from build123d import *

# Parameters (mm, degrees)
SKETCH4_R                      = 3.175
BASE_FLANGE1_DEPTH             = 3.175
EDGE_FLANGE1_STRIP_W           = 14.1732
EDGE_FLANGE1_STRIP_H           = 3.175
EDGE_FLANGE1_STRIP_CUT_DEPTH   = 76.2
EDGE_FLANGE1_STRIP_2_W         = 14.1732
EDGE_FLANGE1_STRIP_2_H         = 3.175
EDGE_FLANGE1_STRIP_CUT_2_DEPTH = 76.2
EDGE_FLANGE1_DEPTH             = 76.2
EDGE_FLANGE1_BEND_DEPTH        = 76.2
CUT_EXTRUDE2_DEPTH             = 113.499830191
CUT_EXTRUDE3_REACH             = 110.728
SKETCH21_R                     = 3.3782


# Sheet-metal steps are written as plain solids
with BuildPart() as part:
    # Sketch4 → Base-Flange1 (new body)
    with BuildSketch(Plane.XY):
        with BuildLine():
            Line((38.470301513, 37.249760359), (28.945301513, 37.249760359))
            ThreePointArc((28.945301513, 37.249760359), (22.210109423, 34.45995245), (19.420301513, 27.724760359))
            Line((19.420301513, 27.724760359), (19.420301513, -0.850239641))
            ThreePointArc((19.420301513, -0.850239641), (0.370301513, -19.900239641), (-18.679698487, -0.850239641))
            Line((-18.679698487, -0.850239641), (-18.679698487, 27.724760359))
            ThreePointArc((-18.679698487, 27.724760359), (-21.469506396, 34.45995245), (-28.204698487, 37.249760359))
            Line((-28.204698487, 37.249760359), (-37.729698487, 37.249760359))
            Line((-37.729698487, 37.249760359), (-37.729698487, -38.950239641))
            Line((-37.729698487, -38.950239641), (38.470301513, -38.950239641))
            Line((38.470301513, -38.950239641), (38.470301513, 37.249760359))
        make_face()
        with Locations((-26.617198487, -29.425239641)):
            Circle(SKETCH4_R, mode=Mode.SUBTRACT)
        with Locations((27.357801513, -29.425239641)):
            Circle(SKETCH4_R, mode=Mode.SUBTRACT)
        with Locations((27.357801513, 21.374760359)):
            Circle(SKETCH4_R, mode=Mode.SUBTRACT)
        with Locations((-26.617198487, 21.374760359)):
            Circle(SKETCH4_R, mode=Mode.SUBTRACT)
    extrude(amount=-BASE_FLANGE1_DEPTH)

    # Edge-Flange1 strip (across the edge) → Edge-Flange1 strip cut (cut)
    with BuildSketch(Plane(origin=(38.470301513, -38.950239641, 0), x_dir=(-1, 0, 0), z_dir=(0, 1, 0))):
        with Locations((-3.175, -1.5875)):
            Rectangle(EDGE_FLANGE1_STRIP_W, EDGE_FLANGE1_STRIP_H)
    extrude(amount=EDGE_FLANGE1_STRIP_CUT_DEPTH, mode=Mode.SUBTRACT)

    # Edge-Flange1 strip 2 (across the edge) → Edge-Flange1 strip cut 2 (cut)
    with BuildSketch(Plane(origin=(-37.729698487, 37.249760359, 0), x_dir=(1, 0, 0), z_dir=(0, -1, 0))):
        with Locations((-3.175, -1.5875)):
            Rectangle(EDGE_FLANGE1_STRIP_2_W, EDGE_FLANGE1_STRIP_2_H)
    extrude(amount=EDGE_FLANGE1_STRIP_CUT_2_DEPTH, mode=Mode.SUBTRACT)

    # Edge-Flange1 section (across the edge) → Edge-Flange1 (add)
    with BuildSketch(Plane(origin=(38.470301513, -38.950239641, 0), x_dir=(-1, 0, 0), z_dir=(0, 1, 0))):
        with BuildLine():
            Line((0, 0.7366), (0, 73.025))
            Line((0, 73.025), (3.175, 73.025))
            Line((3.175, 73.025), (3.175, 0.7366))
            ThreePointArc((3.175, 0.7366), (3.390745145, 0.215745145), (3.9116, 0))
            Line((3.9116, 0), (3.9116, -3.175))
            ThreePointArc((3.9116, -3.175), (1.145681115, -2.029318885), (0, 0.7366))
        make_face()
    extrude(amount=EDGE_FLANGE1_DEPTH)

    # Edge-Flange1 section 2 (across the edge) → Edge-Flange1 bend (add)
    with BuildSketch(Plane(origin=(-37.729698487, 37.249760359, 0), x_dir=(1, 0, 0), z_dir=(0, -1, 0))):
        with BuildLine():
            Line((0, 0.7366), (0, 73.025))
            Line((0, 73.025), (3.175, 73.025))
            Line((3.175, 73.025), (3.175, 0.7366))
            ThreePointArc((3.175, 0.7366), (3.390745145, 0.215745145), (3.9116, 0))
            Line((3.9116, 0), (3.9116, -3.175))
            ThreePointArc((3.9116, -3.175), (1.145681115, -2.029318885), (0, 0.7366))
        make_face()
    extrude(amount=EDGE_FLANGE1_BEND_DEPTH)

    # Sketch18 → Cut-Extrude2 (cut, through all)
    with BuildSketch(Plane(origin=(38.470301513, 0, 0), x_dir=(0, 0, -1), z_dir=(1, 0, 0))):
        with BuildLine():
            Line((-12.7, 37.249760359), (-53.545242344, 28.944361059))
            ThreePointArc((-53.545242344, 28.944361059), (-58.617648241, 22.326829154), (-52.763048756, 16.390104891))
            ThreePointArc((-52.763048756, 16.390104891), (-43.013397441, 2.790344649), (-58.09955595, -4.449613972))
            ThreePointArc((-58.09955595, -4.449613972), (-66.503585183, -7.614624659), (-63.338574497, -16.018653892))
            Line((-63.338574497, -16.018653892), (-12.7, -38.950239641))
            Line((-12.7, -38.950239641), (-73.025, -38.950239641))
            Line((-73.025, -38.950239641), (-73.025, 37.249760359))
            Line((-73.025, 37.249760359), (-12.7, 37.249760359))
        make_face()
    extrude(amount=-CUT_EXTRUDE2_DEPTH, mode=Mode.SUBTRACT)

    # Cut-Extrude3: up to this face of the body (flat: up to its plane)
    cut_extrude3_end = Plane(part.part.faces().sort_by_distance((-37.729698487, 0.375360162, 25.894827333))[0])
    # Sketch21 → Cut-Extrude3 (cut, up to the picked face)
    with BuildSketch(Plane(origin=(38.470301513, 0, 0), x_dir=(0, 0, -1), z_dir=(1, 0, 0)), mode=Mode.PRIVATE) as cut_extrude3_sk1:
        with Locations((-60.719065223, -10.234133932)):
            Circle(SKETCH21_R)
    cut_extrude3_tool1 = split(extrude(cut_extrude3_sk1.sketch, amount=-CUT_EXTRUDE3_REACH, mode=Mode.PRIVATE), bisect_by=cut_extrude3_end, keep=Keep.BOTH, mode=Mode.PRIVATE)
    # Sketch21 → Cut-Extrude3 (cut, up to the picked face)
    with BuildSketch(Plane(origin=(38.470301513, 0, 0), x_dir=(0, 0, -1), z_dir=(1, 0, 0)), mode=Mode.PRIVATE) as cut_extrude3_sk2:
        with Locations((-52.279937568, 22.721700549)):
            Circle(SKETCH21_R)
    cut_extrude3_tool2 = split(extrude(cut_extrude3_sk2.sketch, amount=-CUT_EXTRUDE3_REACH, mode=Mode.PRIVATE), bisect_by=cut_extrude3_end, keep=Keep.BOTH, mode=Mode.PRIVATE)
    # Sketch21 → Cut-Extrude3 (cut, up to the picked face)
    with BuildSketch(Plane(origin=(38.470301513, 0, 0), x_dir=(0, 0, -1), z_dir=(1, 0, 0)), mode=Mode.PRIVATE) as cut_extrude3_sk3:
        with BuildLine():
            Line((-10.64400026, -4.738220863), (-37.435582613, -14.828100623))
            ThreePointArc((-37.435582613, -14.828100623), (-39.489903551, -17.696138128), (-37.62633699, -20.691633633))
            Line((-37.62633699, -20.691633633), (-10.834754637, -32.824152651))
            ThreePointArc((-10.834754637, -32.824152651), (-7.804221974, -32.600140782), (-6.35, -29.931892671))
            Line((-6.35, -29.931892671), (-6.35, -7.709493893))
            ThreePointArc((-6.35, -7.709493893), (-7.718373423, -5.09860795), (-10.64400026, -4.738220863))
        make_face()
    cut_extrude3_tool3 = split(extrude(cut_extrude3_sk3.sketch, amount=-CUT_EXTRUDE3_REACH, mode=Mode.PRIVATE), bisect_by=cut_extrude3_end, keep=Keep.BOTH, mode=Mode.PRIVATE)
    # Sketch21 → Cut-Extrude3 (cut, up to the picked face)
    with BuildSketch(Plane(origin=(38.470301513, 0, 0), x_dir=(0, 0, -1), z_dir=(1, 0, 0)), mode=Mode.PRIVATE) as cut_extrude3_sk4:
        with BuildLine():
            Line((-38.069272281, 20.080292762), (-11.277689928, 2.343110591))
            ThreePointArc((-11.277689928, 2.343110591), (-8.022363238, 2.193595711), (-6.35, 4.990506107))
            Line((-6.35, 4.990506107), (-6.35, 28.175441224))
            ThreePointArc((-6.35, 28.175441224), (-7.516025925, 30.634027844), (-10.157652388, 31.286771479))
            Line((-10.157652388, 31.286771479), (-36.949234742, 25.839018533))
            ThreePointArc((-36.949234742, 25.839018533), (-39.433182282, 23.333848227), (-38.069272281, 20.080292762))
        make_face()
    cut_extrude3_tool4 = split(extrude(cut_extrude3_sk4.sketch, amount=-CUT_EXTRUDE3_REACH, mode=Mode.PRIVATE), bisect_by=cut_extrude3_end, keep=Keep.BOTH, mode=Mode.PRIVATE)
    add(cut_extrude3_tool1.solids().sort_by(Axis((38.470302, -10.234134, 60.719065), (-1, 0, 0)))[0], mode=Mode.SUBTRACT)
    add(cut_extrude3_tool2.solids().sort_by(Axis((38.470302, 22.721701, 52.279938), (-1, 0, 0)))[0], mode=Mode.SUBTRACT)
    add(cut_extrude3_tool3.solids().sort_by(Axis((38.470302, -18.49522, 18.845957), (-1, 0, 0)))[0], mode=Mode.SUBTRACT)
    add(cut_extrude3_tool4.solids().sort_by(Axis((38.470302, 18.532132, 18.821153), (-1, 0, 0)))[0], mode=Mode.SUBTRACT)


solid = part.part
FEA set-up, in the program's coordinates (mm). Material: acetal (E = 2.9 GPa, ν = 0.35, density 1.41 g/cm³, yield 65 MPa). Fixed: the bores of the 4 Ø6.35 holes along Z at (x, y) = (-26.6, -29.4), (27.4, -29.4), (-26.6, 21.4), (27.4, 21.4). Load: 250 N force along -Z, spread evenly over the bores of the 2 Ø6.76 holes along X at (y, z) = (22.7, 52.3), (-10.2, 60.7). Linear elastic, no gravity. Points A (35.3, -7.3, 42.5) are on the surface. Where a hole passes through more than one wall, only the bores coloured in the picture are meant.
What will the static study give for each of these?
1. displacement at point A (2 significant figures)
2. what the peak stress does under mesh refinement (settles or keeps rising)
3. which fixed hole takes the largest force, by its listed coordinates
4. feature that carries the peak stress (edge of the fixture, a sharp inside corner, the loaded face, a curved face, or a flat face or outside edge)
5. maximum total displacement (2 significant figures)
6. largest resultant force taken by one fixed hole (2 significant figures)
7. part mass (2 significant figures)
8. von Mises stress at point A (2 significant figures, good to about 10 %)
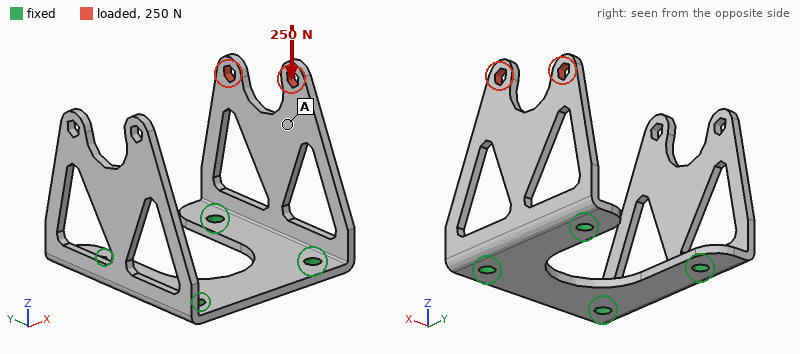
0.88 mm
keeps rising
(27.4, 21.4)
edge of the fixture
1.4 mm
170 N
36 g
2.8 MPa
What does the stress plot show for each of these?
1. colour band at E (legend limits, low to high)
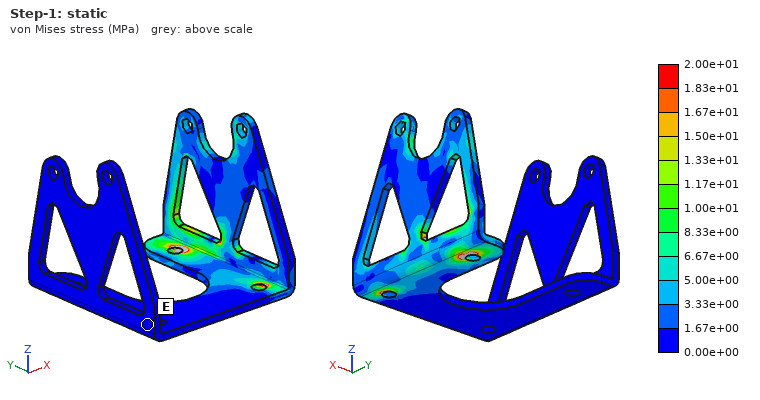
0.00e+00 to 1.67e+00 MPa
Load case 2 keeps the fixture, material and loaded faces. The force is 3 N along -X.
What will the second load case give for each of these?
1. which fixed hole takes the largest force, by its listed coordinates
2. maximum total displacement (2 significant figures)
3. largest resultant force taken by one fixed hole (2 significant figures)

(27.4, 21.4)
1.4 mm
1.8 N
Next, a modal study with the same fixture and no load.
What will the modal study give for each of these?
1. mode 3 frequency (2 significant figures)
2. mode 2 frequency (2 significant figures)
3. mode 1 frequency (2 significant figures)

410 Hz
160 Hz
150 Hz
